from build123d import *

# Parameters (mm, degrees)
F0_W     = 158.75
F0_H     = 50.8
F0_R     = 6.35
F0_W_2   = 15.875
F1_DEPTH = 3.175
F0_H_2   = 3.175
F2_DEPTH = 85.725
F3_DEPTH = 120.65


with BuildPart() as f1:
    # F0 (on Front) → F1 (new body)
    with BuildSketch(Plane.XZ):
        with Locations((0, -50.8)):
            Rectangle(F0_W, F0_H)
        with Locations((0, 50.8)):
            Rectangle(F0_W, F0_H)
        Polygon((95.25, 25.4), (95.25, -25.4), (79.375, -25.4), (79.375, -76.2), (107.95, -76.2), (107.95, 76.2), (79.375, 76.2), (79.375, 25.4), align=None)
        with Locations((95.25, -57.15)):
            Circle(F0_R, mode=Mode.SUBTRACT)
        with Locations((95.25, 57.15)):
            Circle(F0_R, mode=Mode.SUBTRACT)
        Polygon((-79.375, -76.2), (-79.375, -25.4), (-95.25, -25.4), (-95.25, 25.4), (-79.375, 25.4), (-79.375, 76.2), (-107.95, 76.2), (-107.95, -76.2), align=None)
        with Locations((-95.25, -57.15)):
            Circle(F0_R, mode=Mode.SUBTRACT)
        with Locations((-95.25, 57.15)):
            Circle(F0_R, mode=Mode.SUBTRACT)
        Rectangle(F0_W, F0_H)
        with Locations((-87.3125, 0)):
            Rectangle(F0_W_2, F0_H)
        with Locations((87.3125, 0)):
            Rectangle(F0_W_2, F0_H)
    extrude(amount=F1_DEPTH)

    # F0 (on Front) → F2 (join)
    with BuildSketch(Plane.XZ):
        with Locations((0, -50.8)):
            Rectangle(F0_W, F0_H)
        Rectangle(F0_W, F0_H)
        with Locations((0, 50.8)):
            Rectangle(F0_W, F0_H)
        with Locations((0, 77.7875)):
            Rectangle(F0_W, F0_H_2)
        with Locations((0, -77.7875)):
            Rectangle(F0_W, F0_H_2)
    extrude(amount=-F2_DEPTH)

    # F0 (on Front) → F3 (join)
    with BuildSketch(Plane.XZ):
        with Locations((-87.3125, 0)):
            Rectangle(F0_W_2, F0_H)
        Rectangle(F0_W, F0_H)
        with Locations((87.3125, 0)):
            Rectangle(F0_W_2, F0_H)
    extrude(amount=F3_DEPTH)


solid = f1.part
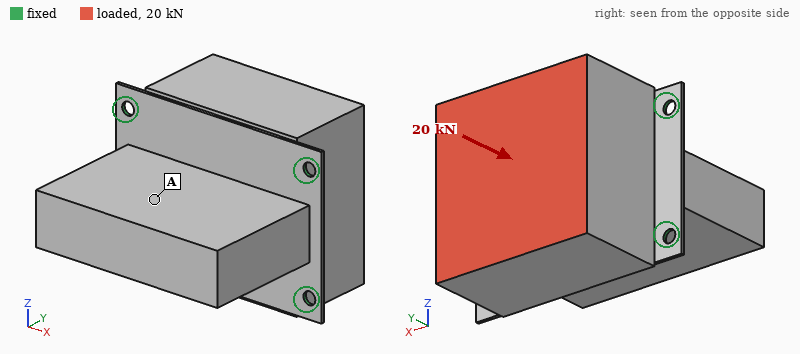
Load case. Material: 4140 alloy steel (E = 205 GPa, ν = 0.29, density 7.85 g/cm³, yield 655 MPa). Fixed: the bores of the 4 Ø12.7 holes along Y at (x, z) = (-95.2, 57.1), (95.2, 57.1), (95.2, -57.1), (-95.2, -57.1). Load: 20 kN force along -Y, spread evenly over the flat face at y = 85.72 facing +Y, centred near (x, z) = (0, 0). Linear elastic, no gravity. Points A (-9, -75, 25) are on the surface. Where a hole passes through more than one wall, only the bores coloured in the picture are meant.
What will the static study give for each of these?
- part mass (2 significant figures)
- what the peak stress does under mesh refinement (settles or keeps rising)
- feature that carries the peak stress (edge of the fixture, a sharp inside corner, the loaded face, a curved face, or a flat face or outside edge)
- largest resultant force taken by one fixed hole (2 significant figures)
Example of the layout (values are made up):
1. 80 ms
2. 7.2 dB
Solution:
1. 27 kg
2. keeps rising
3. edge of the fixture
4. 5.7 kN
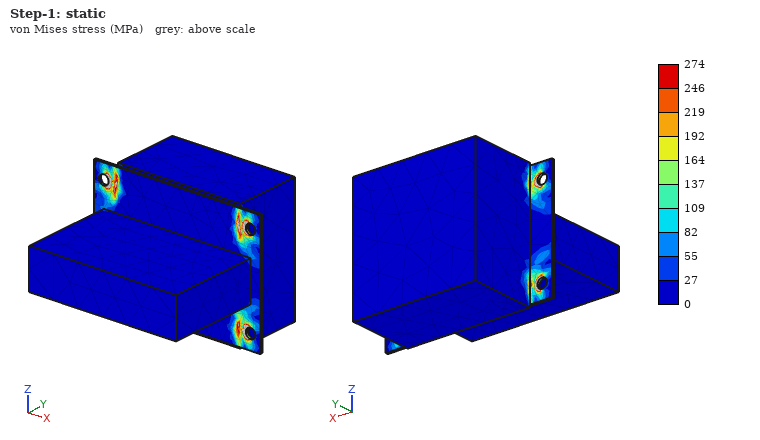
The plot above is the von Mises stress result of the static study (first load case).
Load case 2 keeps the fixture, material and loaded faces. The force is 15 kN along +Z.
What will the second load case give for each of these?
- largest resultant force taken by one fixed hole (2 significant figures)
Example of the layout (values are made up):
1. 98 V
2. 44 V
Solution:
1. 7.8 kN
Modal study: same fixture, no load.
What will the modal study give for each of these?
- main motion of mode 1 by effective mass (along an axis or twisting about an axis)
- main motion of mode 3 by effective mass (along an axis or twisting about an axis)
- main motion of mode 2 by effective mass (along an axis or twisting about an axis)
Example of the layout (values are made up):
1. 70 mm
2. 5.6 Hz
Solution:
1. twisting about X
2. twisting about Z
3. along Y
